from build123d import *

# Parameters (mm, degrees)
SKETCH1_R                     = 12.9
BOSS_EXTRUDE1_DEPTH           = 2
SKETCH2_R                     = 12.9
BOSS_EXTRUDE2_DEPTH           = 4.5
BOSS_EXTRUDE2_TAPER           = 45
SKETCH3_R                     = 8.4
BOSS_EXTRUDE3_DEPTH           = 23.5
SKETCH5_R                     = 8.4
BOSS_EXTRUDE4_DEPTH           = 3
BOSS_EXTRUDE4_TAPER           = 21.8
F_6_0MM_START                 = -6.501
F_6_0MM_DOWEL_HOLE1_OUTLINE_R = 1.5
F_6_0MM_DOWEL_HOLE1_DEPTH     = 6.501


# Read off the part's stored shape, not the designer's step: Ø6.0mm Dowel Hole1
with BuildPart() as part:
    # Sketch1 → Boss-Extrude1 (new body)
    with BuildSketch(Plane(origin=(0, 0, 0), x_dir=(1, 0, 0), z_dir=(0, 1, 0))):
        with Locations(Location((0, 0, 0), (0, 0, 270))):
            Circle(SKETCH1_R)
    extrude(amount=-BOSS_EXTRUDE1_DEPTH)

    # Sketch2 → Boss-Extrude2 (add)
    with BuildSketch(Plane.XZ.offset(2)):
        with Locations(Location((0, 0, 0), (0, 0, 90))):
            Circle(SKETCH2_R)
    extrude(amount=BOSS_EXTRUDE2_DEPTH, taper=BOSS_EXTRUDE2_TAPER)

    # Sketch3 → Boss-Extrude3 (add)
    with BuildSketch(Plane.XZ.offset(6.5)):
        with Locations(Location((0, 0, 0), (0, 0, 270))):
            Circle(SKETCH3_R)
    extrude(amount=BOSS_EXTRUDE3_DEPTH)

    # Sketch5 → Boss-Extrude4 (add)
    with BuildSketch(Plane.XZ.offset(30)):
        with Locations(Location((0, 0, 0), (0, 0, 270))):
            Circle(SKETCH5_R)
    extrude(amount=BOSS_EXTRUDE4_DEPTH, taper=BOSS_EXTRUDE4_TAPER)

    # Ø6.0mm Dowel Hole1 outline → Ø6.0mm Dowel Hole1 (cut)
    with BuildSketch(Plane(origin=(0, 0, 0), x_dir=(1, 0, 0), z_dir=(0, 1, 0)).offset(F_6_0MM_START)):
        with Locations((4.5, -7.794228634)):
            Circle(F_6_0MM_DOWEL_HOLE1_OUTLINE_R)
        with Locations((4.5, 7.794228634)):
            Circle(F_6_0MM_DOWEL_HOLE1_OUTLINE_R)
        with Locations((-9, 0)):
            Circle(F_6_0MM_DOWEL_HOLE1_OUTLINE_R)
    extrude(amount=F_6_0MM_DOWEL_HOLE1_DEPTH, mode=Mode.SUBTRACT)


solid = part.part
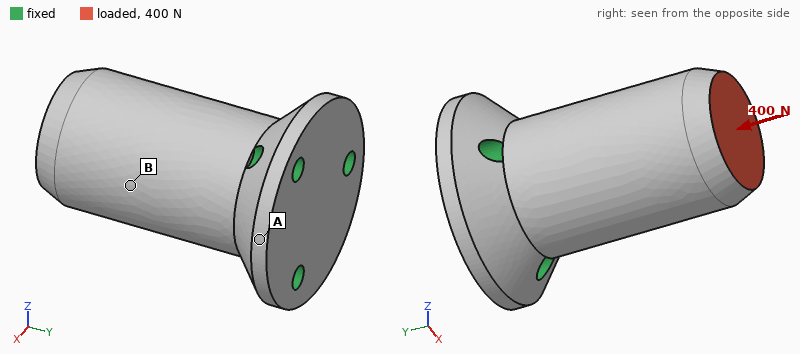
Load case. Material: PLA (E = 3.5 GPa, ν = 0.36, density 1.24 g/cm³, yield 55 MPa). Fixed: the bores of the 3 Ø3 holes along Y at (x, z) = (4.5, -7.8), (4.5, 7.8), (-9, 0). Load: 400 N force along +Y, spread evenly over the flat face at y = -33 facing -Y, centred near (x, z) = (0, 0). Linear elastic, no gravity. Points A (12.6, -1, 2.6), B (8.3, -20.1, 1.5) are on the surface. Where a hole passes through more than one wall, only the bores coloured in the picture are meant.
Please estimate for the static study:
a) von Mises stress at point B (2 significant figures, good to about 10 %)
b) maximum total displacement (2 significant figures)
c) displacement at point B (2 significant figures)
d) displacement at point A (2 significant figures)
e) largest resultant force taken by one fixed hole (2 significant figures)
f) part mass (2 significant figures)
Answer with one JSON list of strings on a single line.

["1.8 MPa", "20 µm", "12 µm", "5.7 µm", "140 N", "10 g"]
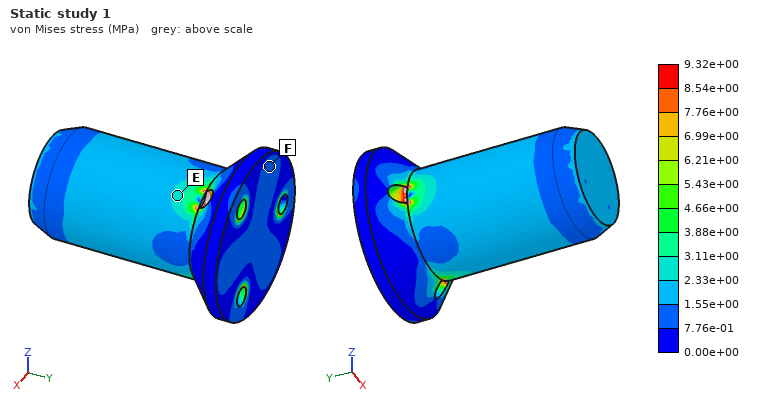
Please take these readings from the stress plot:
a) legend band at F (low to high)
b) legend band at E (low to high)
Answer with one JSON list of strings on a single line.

["7.76e-01 to 1.55e+00 MPa", "2.33e+00 to 3.11e+00 MPa"]
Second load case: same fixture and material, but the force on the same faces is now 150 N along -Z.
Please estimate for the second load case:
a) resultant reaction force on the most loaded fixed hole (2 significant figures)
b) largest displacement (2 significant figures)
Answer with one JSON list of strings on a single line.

["270 N", "0.13 mm"]
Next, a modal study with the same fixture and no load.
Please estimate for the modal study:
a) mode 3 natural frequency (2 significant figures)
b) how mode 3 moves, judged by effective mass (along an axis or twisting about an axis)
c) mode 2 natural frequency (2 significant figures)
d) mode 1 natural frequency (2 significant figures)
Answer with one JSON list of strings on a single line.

["9200 Hz", "twisting about Y", "3700 Hz", "3700 Hz"]
